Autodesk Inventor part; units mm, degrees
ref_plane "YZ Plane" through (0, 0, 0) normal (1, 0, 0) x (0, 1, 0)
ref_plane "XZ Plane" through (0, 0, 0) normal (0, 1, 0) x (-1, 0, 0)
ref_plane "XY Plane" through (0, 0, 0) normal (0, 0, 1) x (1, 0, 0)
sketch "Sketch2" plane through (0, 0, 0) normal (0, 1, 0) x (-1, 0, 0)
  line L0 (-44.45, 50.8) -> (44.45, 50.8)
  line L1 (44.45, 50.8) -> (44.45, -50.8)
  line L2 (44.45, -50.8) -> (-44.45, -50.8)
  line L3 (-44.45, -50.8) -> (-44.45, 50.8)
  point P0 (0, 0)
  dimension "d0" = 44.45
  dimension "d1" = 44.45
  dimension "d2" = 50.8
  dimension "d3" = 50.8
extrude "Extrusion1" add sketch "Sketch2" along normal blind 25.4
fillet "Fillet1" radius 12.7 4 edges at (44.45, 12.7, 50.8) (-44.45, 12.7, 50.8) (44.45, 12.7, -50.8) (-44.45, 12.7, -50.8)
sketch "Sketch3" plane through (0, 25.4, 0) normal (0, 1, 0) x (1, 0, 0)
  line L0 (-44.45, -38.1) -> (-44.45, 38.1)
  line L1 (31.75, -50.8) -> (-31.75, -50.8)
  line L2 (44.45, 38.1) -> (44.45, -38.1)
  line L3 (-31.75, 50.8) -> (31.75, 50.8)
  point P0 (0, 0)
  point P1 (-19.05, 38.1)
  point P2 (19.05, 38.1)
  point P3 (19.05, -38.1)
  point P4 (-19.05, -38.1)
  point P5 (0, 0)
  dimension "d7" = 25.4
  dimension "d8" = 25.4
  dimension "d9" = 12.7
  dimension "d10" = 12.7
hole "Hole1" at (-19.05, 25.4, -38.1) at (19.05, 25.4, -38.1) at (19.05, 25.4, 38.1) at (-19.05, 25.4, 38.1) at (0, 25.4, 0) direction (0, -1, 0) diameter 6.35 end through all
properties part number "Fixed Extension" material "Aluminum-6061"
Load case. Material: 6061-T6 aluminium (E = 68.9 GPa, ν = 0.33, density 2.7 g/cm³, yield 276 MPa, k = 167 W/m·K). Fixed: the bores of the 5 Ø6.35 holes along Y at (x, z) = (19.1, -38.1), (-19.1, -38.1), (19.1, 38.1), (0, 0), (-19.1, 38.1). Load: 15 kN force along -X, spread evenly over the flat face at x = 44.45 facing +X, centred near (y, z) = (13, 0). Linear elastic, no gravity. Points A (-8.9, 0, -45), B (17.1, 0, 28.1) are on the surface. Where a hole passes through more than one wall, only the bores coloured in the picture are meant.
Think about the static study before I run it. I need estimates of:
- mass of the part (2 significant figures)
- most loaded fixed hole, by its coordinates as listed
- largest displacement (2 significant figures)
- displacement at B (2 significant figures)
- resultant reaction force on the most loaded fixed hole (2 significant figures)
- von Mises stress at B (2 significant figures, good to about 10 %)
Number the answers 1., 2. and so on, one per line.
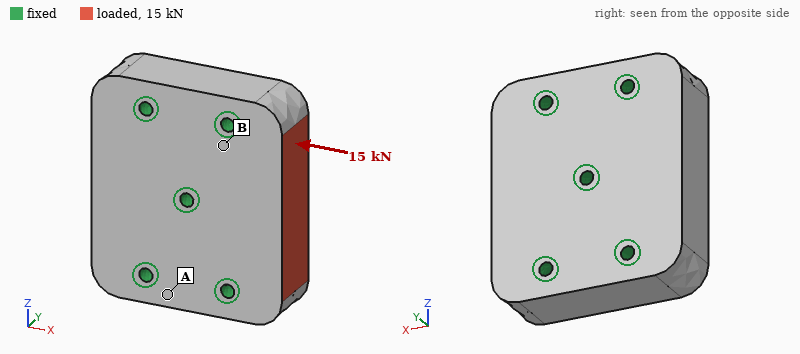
1. 600 g
2. (0, 0)
3. 5.0 µm
4. 1.4 µm
5. 5.1 kN
6. 4.4 MPa
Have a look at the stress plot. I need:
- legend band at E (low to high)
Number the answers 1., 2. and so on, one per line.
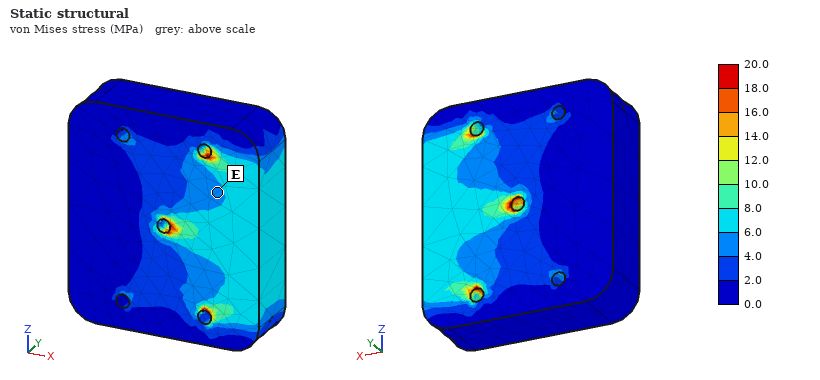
1. 4.0 to 6.0 MPa
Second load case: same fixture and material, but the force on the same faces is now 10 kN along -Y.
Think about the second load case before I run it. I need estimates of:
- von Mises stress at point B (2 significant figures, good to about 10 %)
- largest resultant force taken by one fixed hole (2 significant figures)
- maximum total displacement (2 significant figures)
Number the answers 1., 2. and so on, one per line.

1. 17 MPa
2. 4.9 kN
3. 29 µm
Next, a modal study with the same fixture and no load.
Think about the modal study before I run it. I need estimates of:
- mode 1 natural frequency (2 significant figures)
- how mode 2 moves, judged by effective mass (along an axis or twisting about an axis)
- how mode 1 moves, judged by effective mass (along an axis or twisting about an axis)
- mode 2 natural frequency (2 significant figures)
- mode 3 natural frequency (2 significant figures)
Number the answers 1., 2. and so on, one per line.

1. 13 kHz
2. along Y
3. twisting about Z
4. 13 kHz
5. 21 kHz
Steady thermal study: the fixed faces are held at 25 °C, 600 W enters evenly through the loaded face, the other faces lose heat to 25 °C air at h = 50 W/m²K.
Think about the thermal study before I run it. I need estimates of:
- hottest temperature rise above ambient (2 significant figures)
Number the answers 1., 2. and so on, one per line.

1. 60 K
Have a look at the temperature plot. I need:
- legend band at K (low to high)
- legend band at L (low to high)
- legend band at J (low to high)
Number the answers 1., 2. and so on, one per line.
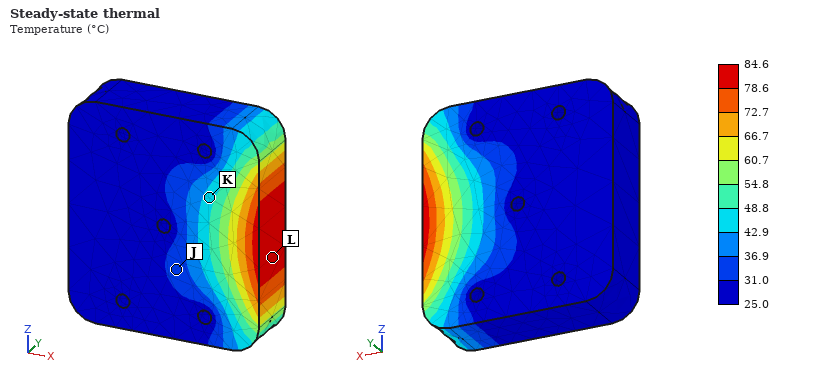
1. 42.9 to 48.8 °C
2. 78.6 to 84.6 °C
3. 31.0 to 36.9 °C
